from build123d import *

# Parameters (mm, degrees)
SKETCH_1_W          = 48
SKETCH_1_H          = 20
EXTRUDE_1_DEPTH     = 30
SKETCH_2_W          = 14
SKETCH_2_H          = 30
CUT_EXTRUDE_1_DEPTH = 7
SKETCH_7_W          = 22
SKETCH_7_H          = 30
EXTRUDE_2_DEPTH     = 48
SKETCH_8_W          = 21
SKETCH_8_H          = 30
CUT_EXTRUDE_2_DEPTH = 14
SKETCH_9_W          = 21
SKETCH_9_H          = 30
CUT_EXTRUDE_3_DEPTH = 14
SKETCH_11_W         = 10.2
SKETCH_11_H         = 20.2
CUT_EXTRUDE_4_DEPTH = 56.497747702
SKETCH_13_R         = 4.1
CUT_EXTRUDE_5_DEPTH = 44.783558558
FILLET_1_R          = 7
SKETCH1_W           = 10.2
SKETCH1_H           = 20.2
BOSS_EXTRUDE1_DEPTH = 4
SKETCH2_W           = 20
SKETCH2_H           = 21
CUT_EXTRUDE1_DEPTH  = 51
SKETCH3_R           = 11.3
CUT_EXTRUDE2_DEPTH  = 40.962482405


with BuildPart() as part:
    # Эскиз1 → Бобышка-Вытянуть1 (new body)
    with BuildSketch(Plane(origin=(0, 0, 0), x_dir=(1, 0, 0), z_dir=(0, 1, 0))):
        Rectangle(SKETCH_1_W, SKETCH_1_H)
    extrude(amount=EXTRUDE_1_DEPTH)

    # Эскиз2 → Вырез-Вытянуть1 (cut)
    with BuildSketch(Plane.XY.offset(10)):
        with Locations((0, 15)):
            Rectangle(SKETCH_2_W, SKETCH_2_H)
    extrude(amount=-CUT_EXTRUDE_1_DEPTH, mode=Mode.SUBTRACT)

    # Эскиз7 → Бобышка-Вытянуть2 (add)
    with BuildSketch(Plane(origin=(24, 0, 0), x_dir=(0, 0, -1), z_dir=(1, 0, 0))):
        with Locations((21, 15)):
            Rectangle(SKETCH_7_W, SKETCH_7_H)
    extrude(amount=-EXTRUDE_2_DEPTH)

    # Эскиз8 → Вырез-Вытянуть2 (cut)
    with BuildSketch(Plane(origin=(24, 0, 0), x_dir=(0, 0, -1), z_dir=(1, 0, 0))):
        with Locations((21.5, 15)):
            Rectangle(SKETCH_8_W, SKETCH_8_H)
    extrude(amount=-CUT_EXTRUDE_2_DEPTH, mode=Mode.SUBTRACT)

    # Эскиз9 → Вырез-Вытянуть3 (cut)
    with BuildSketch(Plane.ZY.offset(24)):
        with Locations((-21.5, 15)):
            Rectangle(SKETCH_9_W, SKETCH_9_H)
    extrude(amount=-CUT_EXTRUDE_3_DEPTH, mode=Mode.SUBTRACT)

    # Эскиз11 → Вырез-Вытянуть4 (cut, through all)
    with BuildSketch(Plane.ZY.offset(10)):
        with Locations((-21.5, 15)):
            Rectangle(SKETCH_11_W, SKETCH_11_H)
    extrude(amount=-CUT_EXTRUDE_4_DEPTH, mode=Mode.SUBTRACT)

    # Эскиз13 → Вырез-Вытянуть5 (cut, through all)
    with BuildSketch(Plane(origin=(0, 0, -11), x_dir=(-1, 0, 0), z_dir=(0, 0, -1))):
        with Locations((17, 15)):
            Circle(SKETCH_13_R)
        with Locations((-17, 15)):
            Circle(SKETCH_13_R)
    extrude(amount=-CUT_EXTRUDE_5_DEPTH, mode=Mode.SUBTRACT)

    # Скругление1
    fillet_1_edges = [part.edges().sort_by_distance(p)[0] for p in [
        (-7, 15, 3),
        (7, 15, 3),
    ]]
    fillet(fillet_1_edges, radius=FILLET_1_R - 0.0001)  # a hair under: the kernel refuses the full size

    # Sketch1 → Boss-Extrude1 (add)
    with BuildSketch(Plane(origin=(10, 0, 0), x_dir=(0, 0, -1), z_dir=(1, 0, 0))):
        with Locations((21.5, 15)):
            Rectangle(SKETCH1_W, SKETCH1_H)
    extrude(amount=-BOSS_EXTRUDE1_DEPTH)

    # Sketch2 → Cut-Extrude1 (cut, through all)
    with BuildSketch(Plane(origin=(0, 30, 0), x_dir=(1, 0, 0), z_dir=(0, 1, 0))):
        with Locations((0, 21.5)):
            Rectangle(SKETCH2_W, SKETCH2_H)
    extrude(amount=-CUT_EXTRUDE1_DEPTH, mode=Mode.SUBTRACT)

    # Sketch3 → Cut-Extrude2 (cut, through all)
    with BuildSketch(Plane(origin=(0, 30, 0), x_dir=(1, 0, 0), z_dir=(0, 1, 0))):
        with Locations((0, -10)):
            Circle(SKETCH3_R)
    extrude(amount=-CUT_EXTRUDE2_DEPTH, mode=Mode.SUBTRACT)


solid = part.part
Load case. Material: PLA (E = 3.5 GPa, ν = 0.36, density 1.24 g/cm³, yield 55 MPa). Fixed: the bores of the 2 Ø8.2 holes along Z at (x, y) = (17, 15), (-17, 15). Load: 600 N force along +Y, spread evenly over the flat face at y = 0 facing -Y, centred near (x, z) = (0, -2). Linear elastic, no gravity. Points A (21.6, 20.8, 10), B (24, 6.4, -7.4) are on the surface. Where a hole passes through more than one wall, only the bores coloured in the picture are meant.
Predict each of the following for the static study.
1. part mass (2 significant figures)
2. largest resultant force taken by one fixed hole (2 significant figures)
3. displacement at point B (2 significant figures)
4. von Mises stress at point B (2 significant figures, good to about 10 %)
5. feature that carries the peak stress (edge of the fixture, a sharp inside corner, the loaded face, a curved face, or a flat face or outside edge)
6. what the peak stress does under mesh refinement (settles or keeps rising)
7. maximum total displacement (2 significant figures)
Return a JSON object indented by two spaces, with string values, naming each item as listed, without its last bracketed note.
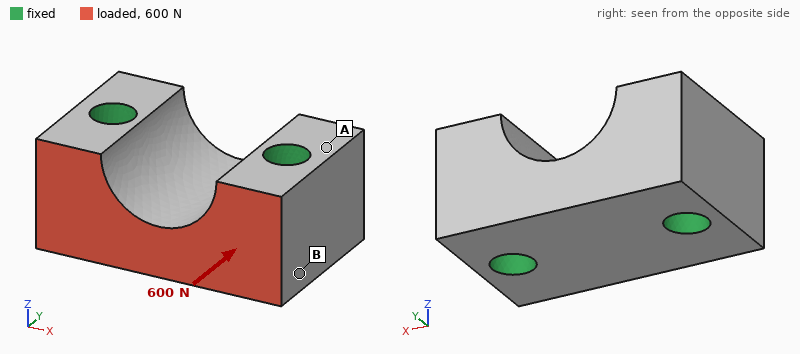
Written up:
{
  "part mass": "27 g",
  "largest resultant force taken by one fixed hole": "300 N",
  "displacement at point B": "1.7 µm",
  "von Mises stress at point B": "0.54 MPa",
  "feature that carries the peak stress": "edge of the fixture",
  "what the peak stress does under mesh refinement": "keeps rising",
  "maximum total displacement": "5.8 µm"
}
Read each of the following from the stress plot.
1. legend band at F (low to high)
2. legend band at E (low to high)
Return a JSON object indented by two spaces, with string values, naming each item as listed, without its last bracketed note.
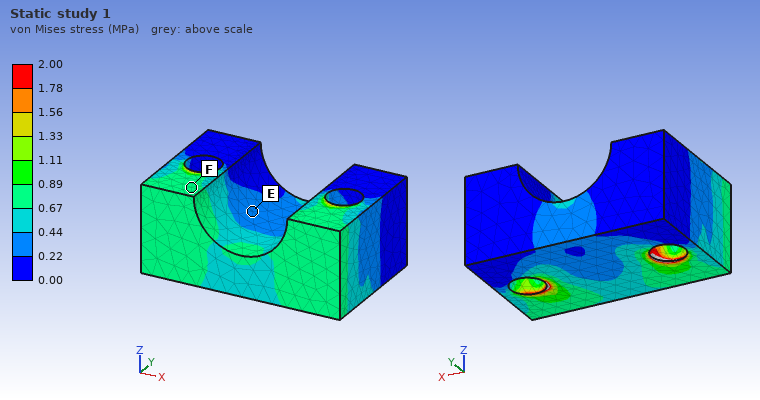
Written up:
{
  "legend band at F": "0.67 to 0.89 MPa",
  "legend band at E": "0.22 to 0.44 MPa"
}
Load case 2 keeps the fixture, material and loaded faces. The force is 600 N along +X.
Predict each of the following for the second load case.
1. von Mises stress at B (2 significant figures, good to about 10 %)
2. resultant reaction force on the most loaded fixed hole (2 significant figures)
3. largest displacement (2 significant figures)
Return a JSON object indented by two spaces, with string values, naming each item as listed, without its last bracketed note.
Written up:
{
  "von Mises stress at B": "1.4 MPa",
  "resultant reaction force on the most loaded fixed hole": "340 N",
  "largest displacement": "18 µm"
}
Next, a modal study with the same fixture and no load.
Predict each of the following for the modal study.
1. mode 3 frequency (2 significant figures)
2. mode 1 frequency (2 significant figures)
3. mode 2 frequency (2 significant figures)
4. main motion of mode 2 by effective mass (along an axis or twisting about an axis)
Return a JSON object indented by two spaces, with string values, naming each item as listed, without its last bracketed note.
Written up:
{
  "mode 3 frequency": "15 kHz",
  "mode 1 frequency": "12 kHz",
  "mode 2 frequency": "13 kHz",
  "main motion of mode 2 by effective mass": "along Z"
}
